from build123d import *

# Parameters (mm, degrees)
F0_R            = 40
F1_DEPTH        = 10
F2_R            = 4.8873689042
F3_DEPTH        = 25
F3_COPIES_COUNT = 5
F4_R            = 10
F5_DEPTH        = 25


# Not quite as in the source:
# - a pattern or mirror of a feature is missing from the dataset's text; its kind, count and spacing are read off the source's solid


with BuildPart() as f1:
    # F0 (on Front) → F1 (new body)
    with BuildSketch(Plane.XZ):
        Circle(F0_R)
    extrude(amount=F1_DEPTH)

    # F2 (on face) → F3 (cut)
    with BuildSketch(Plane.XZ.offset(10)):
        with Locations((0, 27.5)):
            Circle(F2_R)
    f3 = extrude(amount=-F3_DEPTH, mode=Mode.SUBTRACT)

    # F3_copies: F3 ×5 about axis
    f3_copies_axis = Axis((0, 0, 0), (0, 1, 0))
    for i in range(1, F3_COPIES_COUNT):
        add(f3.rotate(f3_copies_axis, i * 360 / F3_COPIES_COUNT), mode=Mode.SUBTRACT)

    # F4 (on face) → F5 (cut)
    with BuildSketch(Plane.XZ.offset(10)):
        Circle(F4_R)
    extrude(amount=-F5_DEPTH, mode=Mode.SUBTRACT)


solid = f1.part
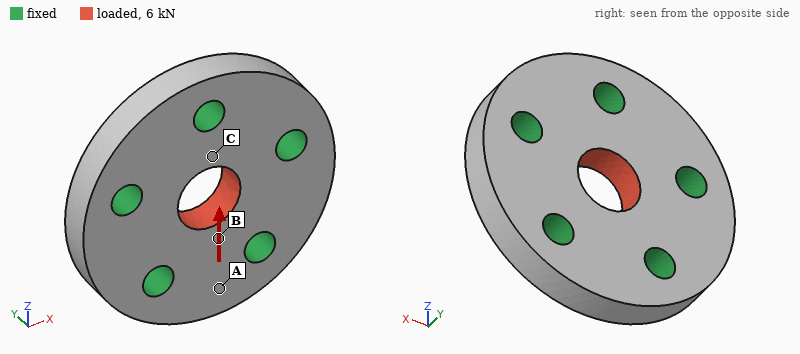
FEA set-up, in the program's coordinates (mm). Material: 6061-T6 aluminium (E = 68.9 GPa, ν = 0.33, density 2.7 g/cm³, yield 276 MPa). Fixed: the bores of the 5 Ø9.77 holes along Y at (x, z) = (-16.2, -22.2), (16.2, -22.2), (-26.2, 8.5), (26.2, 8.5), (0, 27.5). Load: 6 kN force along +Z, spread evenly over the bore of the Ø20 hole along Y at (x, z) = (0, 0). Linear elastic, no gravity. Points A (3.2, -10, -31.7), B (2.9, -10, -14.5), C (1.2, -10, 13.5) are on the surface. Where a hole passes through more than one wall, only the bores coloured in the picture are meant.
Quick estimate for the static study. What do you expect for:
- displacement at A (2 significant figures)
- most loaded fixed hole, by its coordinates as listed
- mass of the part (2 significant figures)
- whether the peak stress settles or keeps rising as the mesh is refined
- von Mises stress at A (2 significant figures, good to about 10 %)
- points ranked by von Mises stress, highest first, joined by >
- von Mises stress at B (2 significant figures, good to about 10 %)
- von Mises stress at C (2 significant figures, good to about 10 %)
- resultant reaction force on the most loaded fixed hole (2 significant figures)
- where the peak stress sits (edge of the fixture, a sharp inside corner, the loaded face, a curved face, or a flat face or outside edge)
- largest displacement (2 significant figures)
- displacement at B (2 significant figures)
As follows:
0.80 µm
(0, 27.5)
120 g
keeps rising
2.3 MPa
C > B > A
7.6 MPa
11 MPa
1.8 kN
edge of the fixture
2.4 µm
1.7 µm
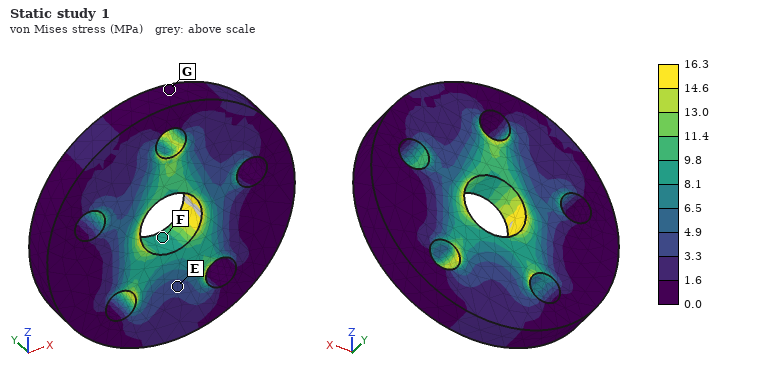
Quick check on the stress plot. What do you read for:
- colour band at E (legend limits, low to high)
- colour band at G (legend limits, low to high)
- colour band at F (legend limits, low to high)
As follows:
3.3 to 4.9 MPa
0.0 to 1.6 MPa
8.1 to 9.8 MPa
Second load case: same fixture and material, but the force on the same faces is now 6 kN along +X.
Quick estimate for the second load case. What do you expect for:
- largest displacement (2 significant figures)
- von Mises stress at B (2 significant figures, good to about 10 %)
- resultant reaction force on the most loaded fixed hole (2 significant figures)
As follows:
2.4 µm
7.7 MPa
1.7 kN
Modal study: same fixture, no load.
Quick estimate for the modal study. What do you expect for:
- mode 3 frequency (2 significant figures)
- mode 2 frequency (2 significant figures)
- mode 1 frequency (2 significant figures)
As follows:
28 kHz
27 kHz
27 kHz
